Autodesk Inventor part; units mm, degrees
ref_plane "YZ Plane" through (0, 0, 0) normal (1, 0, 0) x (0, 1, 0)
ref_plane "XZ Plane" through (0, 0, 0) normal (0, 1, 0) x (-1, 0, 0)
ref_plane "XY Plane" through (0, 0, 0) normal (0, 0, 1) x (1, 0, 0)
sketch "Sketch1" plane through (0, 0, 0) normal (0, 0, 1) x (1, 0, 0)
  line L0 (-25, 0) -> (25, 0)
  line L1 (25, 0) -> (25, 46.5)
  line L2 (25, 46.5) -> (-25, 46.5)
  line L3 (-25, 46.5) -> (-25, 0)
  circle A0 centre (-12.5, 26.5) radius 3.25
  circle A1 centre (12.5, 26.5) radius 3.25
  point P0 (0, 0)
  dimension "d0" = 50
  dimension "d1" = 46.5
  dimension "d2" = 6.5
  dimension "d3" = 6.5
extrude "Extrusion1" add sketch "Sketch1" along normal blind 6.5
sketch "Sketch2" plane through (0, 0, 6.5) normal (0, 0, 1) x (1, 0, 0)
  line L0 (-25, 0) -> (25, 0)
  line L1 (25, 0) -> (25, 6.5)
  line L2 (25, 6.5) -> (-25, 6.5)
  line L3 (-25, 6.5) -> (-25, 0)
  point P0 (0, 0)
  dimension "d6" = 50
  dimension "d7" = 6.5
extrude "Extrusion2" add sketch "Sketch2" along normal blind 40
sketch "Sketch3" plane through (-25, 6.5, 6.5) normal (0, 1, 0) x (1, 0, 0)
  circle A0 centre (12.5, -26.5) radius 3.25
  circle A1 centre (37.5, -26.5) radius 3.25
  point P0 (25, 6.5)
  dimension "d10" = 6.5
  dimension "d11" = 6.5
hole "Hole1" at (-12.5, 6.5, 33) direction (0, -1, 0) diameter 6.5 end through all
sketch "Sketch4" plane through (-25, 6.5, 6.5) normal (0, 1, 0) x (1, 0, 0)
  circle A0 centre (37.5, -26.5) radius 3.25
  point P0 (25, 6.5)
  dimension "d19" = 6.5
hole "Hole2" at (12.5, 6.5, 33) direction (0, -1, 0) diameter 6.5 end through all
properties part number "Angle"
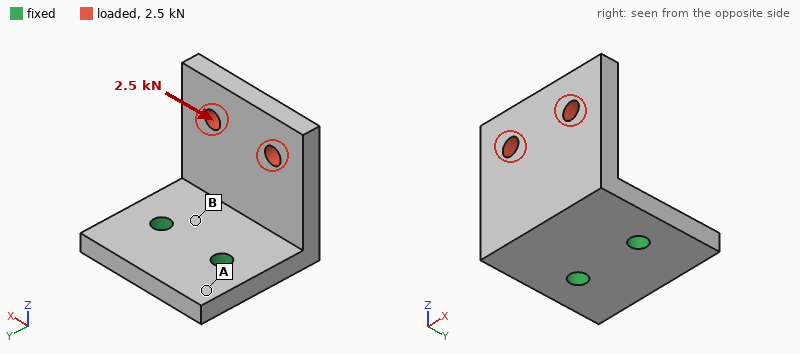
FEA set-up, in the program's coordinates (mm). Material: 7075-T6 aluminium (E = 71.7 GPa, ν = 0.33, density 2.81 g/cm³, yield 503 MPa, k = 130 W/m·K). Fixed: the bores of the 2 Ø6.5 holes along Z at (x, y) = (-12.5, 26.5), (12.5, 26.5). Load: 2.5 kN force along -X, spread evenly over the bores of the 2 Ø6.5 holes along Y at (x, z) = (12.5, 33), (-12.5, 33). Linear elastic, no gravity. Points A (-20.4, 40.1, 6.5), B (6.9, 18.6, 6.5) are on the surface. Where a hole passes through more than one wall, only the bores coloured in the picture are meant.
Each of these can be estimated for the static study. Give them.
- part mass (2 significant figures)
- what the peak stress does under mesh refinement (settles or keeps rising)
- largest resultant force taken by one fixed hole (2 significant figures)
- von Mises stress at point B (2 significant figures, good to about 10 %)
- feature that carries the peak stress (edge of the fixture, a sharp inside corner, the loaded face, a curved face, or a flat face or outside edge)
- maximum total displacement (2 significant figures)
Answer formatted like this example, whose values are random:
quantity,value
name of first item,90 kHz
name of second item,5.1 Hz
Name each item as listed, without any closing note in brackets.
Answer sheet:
quantity,value
part mass,77 g
what the peak stress does under mesh refinement,keeps rising
largest resultant force taken by one fixed hole,3.2 kN
von Mises stress at point B,99 MPa
feature that carries the peak stress,edge of the fixture
maximum total displacement,0.32 mm
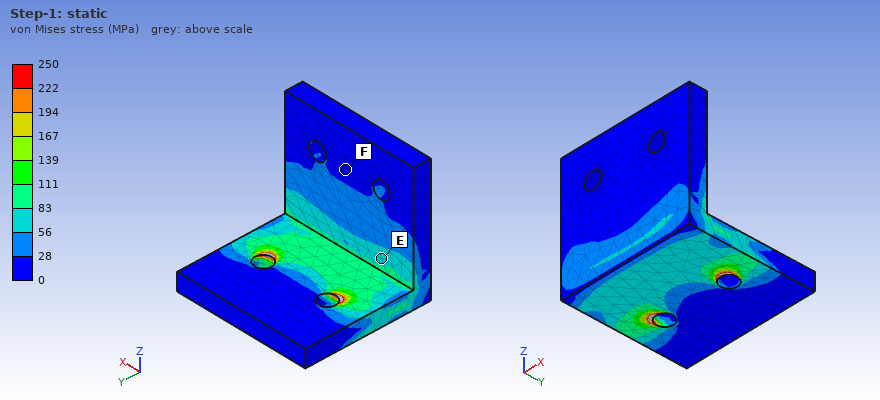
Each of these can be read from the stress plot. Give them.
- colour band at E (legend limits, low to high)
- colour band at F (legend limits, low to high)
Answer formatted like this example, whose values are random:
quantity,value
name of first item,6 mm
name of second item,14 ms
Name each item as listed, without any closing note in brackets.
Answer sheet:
quantity,value
colour band at E,56 to 83 MPa
colour band at F,0 to 28 MPa
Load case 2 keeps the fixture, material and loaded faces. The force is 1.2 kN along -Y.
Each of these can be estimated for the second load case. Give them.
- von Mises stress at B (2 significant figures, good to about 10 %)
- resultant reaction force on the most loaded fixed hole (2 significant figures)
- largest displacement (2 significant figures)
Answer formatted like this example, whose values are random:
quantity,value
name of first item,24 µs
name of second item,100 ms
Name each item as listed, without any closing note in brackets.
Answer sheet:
quantity,value
von Mises stress at B,94 MPa
resultant reaction force on the most loaded fixed hole,630 N
largest displacement,0.59 mm
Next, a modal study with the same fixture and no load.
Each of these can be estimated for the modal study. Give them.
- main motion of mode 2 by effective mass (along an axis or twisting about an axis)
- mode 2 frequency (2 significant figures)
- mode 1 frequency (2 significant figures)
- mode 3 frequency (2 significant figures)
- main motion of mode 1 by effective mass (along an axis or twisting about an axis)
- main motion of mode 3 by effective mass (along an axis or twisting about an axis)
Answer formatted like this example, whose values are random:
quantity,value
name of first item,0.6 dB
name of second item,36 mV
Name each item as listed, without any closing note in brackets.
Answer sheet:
quantity,value
main motion of mode 2 by effective mass,along X
mode 2 frequency,3000 Hz
mode 1 frequency,1600 Hz
mode 3 frequency,5200 Hz
main motion of mode 1 by effective mass,along Y
main motion of mode 3 by effective mass,along Z
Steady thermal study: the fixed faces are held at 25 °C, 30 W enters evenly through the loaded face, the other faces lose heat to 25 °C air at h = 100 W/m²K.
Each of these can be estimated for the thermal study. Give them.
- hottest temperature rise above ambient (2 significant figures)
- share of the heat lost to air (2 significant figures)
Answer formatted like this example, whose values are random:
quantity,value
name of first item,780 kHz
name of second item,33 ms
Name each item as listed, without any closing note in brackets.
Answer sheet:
quantity,value
hottest temperature rise above ambient,28 K
share of the heat lost to air,38 %
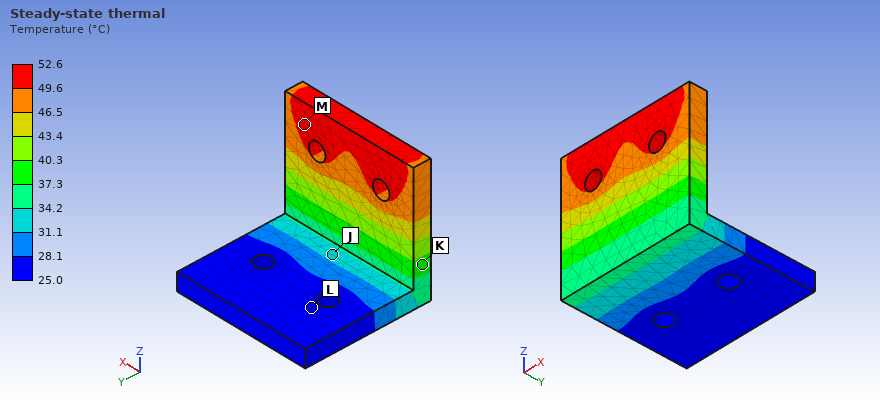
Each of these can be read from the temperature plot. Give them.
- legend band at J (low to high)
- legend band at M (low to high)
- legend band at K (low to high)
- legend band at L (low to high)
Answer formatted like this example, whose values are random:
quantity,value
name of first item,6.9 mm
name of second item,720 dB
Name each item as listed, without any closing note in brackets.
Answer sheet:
quantity,value
legend band at J,31.1 to 34.2 °C
legend band at M,49.6 to 52.6 °C
legend band at K,37.3 to 40.3 °C
legend band at L,25.0 to 28.1 °C
